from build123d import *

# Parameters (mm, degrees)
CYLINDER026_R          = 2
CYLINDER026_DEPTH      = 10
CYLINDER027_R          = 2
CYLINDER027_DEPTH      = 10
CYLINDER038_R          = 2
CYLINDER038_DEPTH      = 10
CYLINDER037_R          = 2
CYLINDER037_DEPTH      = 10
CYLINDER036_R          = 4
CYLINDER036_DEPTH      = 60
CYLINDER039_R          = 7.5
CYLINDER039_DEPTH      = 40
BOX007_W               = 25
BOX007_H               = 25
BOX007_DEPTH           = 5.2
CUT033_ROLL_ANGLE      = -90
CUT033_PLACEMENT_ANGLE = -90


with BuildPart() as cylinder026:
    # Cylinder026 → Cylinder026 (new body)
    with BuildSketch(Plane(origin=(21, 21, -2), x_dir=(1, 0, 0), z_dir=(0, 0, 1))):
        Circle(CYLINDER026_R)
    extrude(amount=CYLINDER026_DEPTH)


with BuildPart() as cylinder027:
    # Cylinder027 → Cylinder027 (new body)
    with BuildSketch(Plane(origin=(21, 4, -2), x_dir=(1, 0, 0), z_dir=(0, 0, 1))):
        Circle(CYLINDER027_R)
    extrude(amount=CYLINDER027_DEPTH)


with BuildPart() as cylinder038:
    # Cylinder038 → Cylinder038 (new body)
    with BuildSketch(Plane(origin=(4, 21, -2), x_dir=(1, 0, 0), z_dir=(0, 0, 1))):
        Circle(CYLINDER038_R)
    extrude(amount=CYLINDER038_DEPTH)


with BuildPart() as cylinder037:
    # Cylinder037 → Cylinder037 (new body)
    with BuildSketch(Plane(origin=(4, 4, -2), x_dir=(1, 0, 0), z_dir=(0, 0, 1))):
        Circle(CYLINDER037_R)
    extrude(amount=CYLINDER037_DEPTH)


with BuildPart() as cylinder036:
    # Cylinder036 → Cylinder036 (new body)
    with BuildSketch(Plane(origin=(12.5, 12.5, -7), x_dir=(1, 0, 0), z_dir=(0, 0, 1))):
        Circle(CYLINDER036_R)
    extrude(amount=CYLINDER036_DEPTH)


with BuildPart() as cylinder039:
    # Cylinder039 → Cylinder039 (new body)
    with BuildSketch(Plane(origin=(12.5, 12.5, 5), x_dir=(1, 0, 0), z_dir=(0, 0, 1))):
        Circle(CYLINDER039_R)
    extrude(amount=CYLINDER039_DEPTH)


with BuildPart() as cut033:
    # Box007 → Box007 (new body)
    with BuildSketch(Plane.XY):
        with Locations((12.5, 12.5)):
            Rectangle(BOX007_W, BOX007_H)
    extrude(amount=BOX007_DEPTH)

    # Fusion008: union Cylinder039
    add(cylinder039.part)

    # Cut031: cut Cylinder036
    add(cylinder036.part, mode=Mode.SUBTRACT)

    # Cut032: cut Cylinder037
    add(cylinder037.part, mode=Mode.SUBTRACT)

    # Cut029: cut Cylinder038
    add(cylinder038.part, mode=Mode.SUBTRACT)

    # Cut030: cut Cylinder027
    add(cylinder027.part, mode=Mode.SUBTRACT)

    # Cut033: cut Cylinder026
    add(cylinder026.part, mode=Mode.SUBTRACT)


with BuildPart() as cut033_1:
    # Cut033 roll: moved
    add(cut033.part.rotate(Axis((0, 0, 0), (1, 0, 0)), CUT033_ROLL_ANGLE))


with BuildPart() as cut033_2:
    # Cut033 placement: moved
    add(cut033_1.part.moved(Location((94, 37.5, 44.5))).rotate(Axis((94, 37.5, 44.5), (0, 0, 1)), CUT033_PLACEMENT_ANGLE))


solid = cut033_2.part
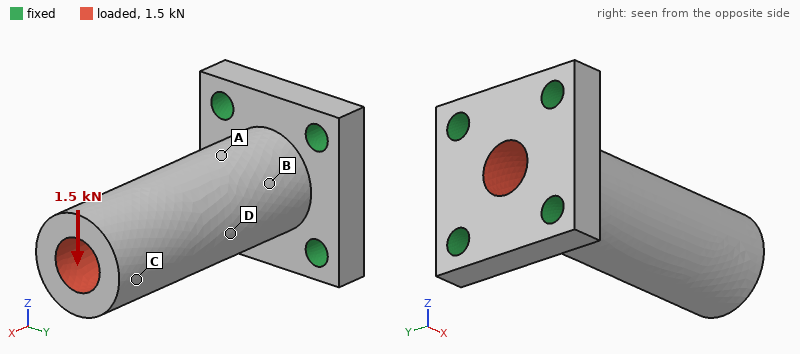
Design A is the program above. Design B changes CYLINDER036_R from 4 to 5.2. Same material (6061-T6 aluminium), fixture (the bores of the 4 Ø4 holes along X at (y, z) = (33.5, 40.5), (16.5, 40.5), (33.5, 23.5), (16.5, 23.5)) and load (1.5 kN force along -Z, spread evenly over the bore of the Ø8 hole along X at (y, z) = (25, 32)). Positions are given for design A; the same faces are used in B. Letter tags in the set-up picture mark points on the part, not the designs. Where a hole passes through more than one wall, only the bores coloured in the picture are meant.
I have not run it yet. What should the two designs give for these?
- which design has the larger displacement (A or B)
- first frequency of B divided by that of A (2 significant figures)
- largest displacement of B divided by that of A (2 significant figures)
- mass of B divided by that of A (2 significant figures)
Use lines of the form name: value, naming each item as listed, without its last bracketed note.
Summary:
which design has the larger displacement: B
first frequency of B divided by that of A: 1.1
largest displacement of B divided by that of A: 1.2
mass of B divided by that of A: 0.80
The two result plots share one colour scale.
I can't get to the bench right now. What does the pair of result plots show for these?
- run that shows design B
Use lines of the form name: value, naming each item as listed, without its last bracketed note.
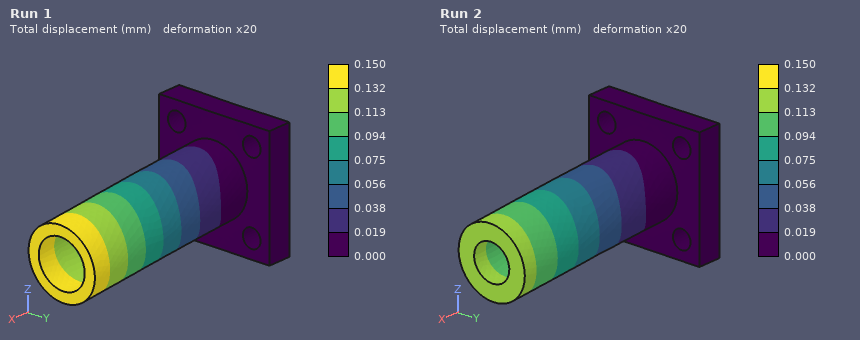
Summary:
run that shows design B: Run 1
